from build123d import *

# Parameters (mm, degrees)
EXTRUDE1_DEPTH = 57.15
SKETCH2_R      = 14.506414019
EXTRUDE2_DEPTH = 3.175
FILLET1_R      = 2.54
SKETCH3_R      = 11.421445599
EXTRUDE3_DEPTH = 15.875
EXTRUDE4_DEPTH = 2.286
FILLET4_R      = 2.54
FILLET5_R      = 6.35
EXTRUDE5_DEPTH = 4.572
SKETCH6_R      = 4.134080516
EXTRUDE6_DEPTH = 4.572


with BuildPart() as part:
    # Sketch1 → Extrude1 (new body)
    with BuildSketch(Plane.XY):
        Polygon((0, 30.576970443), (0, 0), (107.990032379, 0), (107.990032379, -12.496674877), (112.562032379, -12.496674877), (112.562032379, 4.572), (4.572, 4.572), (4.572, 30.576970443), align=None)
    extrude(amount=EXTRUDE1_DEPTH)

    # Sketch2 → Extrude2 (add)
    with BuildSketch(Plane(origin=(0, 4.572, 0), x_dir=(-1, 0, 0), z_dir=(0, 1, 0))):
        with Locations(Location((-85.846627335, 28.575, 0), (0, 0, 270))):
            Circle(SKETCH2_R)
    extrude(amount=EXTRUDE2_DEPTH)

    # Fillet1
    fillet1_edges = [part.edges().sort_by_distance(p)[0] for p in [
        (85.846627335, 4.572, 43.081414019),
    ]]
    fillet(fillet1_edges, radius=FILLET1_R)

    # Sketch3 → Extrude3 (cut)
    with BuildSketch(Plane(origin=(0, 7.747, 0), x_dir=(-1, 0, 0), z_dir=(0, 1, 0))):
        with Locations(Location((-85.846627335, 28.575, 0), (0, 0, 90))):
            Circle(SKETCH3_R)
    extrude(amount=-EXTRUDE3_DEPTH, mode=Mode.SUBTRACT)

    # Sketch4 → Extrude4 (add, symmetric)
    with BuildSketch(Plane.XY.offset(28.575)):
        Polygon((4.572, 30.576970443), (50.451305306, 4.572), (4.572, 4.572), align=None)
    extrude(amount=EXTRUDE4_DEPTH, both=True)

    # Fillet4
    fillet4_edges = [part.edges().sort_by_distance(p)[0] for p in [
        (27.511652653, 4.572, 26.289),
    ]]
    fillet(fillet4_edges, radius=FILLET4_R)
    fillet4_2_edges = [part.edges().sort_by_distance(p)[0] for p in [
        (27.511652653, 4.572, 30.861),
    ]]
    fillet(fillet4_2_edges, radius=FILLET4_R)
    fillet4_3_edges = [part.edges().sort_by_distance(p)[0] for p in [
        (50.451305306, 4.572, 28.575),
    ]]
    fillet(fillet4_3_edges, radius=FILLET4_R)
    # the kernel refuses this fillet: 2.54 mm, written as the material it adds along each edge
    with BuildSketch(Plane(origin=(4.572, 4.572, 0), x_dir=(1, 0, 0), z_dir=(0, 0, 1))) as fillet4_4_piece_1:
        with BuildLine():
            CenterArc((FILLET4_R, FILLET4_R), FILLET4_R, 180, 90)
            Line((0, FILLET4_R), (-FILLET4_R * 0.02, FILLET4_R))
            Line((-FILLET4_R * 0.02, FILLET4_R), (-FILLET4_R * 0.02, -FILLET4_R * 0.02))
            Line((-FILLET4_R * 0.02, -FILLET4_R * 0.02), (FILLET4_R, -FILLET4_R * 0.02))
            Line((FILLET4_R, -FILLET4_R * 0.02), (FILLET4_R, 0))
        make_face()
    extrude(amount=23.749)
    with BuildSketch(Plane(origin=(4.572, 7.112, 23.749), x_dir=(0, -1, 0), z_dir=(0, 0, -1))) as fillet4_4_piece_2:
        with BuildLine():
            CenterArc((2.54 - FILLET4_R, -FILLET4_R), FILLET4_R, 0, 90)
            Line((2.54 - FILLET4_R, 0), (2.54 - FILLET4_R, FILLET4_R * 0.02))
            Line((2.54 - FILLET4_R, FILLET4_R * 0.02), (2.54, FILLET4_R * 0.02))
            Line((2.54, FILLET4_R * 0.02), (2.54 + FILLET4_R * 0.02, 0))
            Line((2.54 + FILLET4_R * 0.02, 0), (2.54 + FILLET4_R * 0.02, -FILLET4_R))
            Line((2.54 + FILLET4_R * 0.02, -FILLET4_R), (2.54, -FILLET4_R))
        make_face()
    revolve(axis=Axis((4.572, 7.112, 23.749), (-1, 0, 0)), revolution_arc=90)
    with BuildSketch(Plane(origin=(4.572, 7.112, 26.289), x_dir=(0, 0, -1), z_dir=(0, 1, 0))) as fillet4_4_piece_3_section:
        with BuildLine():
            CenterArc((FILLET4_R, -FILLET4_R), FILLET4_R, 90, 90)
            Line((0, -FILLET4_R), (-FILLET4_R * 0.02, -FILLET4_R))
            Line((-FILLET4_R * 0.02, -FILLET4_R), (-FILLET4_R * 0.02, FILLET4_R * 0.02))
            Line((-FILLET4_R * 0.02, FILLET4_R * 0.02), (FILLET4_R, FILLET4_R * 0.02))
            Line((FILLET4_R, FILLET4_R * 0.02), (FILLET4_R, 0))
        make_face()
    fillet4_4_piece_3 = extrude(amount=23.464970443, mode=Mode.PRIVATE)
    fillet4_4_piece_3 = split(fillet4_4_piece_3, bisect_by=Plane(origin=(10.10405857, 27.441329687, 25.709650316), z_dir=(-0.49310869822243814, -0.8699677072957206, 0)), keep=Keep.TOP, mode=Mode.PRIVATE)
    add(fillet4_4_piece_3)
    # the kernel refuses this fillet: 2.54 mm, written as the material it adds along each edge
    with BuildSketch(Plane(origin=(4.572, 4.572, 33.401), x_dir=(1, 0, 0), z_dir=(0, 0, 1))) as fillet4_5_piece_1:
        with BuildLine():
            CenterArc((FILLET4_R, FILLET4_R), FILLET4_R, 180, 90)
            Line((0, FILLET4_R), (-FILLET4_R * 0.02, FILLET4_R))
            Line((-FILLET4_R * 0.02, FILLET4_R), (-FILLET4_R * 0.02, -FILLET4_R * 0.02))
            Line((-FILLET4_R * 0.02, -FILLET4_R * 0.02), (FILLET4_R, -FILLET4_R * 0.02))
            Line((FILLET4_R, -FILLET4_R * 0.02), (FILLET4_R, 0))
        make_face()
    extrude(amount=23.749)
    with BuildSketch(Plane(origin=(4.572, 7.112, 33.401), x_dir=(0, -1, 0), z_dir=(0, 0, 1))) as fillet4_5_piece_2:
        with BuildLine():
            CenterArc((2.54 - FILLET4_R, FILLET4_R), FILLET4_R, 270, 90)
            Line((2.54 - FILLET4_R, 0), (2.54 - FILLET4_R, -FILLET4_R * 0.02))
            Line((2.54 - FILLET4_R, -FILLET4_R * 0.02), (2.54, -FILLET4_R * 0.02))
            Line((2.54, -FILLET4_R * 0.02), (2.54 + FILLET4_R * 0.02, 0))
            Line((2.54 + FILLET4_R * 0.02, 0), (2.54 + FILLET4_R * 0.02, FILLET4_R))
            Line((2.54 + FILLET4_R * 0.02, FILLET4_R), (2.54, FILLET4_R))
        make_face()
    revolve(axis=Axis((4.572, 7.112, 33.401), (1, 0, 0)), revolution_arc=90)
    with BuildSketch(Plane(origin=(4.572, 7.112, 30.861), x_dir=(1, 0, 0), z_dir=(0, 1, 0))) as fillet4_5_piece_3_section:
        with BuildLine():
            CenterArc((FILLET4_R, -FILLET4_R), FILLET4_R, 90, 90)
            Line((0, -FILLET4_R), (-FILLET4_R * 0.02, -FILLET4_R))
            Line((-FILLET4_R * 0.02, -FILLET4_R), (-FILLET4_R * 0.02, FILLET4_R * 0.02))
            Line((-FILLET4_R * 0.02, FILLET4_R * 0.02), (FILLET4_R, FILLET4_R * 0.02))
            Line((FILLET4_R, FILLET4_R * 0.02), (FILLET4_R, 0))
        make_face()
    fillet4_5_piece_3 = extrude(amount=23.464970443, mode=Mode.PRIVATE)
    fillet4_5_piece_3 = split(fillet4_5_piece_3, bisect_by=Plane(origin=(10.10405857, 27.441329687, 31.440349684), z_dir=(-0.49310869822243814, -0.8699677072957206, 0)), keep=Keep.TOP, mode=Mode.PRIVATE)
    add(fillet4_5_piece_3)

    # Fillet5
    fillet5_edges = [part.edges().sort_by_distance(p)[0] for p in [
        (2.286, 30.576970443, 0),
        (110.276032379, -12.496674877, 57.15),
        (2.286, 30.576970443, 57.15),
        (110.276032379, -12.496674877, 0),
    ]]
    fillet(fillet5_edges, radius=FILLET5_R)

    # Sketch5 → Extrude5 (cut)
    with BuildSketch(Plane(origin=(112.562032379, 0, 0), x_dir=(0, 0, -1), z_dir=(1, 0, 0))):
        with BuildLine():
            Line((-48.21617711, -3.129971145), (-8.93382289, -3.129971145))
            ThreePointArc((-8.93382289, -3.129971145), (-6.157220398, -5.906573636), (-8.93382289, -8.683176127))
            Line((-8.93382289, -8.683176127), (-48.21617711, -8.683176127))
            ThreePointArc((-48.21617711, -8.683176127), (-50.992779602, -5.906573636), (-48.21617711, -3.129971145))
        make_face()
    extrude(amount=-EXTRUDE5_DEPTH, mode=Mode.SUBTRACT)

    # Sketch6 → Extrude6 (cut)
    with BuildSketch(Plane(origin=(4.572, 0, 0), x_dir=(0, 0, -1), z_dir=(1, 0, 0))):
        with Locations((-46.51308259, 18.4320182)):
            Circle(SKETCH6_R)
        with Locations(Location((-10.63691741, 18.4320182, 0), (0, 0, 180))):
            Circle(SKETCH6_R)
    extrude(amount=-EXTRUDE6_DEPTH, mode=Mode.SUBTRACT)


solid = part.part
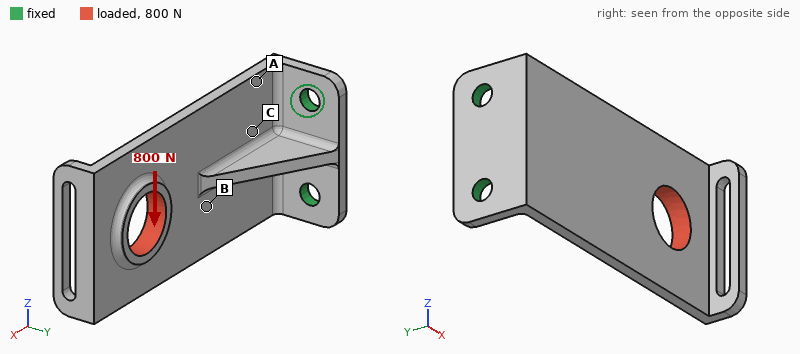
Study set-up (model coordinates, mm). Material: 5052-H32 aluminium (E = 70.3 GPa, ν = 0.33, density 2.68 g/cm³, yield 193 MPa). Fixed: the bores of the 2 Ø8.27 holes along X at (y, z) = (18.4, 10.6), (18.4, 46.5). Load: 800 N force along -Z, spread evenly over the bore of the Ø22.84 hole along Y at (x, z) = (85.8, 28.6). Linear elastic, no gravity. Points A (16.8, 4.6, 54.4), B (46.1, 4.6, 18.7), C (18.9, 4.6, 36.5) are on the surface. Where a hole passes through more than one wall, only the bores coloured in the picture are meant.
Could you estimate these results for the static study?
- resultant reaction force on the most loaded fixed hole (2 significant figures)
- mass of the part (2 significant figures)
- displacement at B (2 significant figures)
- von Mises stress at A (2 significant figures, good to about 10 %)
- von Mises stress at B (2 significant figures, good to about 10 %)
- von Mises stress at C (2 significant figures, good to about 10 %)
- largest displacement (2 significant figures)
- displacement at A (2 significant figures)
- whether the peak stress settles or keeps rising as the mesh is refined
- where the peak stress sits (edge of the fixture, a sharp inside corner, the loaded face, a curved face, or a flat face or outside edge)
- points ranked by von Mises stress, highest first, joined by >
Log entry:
1.9 kN
110 g
0.15 mm
46 MPa
13 MPa
23 MPa
0.40 mm
0.099 mm
keeps rising
edge of the fixture
A > C > B
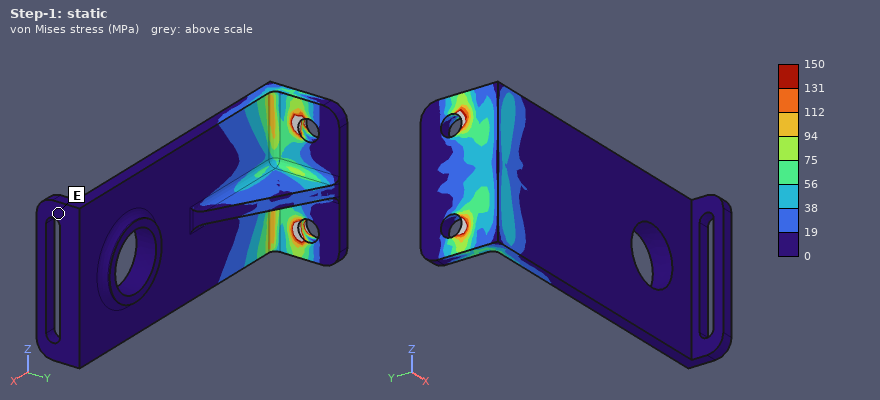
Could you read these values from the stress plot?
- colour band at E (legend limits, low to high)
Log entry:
0 to 19 MPa
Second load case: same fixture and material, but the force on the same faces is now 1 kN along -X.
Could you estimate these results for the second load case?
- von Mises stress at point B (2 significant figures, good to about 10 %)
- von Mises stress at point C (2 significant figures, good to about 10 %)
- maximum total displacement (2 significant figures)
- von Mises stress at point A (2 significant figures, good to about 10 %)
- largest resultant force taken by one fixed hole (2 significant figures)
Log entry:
9.5 MPa
4.5 MPa
72 µm
9.3 MPa
500 N
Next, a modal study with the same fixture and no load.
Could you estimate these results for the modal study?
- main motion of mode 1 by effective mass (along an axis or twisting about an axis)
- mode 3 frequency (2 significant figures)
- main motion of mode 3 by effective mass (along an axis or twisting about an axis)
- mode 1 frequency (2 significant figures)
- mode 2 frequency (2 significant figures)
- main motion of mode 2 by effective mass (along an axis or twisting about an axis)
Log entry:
along Y
1200 Hz
along Z
460 Hz
1100 Hz
along Z
